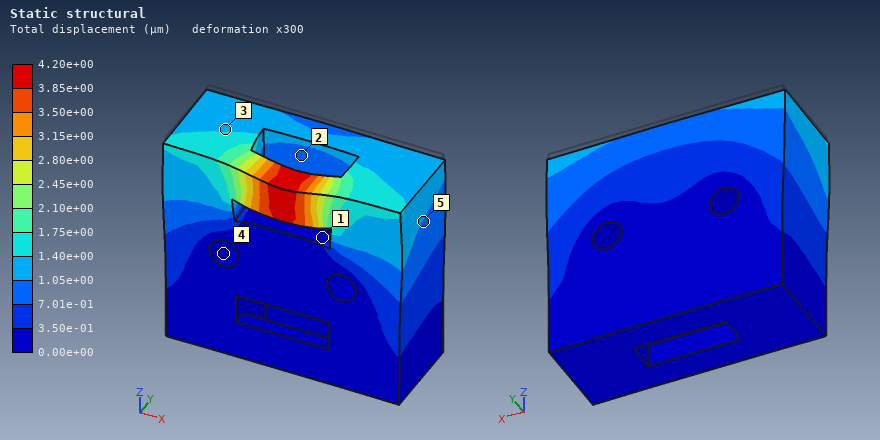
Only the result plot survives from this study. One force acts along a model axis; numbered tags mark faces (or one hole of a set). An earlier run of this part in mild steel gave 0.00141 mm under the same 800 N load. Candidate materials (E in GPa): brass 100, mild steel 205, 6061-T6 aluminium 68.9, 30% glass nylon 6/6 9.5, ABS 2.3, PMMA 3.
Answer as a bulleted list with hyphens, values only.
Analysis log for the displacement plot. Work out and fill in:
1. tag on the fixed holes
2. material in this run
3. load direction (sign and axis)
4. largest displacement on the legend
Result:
- 4
- 6061-T6 aluminium
- -Z
- 4.20e+00 µm
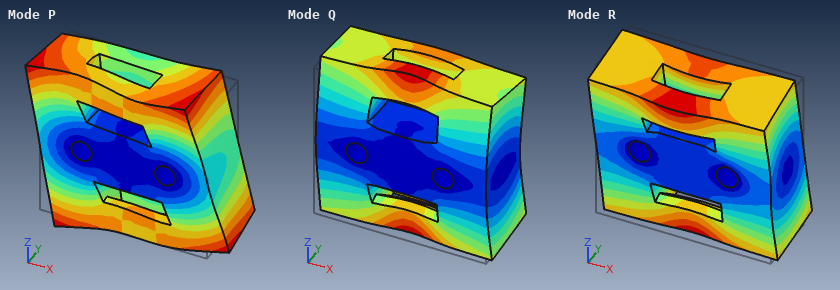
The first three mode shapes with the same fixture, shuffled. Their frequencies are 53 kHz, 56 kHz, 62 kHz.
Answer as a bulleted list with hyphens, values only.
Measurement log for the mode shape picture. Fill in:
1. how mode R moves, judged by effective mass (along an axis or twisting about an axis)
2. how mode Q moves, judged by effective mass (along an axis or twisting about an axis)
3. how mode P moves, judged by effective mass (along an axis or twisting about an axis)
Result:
- twisting about X
- along Y
- twisting about Y
